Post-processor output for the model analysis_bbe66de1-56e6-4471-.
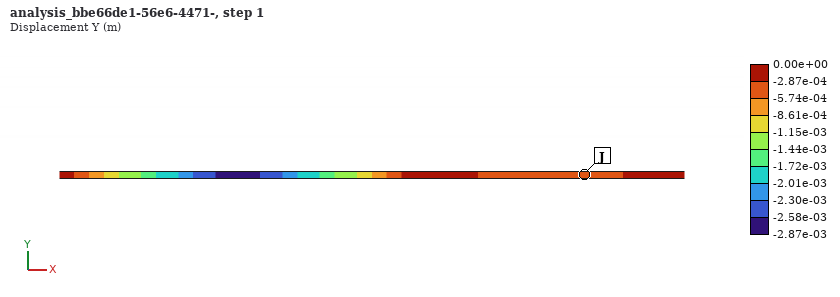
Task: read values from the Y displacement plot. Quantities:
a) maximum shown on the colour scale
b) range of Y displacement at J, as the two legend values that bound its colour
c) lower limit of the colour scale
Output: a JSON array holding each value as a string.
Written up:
["0.00e+00 m", "-5.74e-04 to -2.87e-04 m", "-2.87e-03 m"]
